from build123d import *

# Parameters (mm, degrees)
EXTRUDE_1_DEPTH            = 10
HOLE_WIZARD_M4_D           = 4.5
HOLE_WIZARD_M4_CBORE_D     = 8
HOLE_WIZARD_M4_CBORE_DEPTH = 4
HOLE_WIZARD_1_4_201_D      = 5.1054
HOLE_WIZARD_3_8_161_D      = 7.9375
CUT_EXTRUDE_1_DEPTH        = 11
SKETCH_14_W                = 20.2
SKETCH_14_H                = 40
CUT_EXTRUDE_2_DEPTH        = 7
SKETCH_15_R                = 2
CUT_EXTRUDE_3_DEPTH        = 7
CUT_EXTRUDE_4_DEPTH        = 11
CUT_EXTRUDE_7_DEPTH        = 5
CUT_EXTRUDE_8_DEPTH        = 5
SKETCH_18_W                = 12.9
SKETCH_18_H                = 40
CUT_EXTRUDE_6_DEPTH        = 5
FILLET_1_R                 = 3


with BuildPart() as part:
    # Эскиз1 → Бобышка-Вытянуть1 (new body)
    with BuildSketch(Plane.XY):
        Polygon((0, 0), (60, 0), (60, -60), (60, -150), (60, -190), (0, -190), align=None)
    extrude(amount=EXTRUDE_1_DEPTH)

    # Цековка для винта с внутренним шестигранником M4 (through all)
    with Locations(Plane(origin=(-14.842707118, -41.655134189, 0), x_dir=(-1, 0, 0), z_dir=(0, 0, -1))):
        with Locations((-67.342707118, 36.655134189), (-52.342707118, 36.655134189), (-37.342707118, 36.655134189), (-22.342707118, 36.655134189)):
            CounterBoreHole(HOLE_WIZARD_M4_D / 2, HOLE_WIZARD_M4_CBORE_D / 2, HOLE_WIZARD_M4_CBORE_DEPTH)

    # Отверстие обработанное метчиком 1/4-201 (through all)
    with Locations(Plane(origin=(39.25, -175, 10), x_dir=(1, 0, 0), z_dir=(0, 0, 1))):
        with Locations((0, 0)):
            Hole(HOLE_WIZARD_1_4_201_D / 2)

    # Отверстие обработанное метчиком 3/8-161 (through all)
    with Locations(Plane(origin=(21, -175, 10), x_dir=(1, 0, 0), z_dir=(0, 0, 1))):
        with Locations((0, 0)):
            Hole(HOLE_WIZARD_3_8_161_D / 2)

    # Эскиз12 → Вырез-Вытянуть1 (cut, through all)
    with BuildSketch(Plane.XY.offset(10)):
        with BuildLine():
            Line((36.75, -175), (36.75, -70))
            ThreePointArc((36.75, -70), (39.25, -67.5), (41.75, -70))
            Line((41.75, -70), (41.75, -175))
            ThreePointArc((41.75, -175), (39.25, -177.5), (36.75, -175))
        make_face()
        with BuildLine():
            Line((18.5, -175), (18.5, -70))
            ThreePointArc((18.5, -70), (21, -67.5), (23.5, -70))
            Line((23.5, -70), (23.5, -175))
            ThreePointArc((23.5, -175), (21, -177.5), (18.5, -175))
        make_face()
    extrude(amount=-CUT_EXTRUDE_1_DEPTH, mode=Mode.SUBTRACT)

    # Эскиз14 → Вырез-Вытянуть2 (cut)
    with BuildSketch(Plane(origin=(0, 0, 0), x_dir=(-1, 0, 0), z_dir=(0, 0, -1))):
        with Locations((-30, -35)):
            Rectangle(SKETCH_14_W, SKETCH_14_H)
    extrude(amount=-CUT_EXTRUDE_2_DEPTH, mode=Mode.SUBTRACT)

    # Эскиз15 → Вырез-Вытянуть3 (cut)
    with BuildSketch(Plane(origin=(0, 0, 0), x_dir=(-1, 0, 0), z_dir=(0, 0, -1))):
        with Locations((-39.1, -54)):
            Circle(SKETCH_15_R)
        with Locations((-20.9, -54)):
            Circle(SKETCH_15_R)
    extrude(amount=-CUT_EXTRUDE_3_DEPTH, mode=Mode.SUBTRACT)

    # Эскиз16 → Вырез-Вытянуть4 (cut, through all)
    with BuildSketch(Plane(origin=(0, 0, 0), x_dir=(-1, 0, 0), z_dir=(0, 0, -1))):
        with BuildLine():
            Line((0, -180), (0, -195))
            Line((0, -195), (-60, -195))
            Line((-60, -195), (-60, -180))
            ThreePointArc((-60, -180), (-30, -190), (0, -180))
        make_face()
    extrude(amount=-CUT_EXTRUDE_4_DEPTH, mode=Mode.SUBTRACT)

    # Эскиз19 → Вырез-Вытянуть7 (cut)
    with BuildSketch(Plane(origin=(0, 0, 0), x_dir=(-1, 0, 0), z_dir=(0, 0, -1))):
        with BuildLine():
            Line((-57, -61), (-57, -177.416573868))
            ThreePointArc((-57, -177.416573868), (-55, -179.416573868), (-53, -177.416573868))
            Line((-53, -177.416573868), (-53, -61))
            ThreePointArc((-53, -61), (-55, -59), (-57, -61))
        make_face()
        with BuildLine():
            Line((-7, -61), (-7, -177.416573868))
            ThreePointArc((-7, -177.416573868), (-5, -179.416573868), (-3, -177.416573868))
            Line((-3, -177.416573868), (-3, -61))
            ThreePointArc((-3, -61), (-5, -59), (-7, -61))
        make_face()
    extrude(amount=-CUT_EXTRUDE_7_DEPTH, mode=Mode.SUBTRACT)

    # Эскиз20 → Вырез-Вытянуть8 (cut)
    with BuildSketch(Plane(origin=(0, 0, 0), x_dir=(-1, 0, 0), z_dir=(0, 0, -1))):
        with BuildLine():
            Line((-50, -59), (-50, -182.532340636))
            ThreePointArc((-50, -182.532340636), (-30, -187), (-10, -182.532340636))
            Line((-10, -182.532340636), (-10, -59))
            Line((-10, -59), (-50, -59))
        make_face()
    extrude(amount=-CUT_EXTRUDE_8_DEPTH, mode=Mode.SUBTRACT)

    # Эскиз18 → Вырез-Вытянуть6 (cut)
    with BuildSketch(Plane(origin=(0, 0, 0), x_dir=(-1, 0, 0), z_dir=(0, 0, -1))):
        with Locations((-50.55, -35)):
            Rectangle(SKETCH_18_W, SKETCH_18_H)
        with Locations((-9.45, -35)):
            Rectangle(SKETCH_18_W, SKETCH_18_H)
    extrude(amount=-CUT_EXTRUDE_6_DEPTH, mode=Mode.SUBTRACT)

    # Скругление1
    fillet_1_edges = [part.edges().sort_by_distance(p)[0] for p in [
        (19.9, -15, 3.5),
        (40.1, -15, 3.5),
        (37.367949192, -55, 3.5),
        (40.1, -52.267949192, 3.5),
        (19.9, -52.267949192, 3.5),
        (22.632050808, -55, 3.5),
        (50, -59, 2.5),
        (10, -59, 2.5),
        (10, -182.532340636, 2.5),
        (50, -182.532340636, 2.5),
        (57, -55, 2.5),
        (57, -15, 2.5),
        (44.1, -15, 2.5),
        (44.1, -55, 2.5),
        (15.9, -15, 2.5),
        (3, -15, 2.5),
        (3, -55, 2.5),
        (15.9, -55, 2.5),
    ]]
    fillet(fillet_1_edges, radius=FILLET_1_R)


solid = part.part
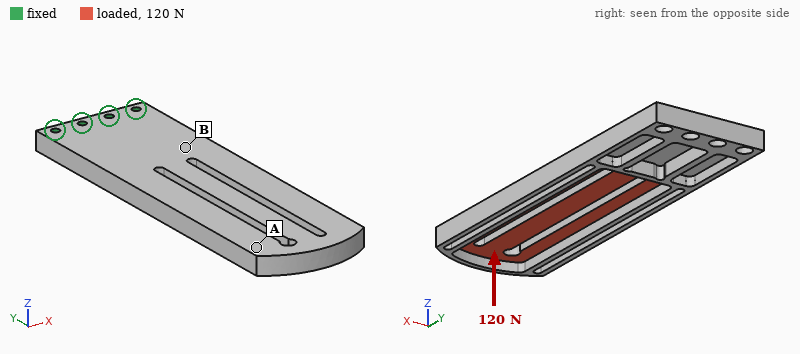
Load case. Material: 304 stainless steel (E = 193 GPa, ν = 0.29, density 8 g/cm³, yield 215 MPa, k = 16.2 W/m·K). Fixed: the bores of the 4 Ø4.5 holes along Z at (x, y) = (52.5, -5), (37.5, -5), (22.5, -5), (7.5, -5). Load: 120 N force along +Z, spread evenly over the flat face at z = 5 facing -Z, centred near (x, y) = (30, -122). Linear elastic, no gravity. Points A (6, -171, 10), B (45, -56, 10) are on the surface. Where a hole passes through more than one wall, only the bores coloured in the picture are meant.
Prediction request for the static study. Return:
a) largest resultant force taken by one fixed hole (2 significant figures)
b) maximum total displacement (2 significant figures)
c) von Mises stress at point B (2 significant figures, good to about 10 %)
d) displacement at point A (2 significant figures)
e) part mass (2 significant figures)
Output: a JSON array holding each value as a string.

["110 N", "0.32 mm", "13 MPa", "0.27 mm", "520 g"]
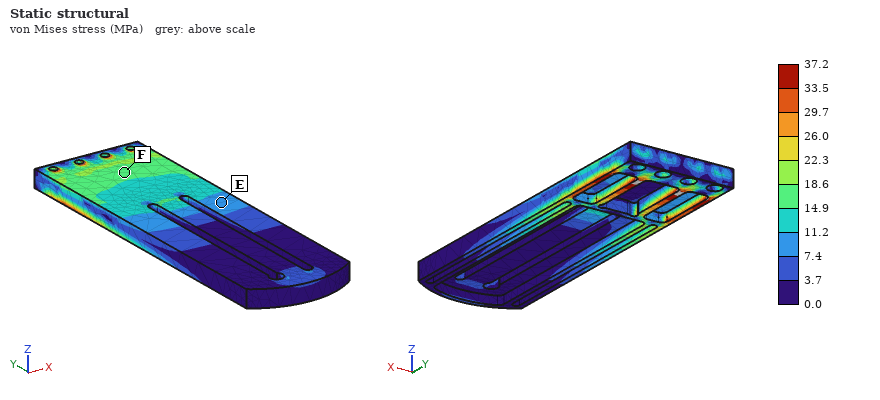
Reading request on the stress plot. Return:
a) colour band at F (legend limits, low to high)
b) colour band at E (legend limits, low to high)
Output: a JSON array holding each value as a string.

["14.9 to 18.6 MPa", "7.4 to 11.2 MPa"]
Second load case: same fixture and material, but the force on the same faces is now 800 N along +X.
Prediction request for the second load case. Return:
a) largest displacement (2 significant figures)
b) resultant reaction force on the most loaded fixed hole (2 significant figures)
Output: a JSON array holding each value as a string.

["0.11 mm", "1.9 kN"]
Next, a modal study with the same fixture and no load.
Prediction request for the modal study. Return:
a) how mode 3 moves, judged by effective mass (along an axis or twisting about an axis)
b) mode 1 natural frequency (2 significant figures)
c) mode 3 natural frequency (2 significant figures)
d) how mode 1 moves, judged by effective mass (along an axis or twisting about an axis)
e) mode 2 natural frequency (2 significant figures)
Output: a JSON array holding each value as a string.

["along X", "210 Hz", "970 Hz", "along Z", "680 Hz"]
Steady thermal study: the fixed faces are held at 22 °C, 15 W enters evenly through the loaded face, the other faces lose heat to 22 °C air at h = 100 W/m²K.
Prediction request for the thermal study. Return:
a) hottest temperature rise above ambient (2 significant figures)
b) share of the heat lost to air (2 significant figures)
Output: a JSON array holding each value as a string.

["21 K", "99 %"]
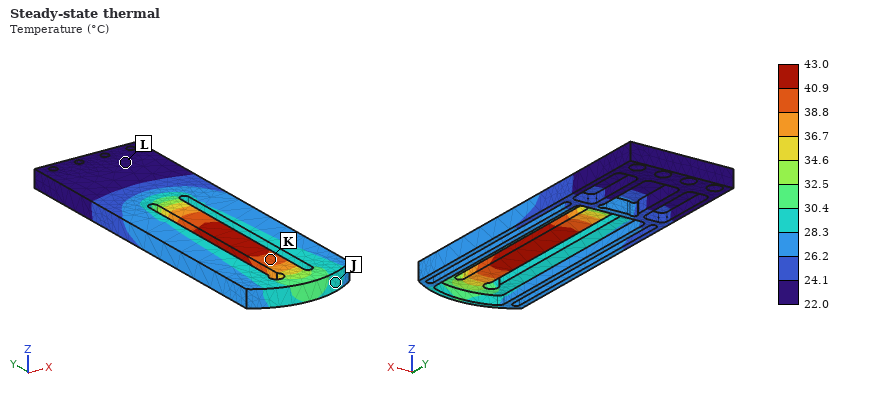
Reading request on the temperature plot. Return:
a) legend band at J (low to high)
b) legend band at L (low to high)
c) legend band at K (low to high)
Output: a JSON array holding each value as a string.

["28.3 to 30.4 °C", "22.0 to 24.1 °C", "38.8 to 40.9 °C"]
